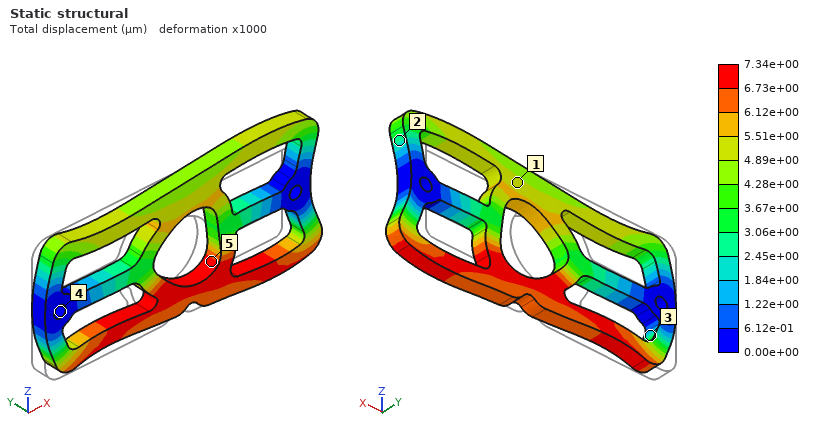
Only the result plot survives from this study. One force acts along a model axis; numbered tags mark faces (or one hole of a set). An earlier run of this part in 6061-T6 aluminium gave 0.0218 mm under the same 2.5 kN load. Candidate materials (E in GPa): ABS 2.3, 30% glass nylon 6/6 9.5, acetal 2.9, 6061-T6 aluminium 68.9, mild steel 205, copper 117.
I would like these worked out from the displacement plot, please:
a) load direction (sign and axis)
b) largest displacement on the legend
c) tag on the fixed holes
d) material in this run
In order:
+X
7.34e+00 µm
4
mild steel
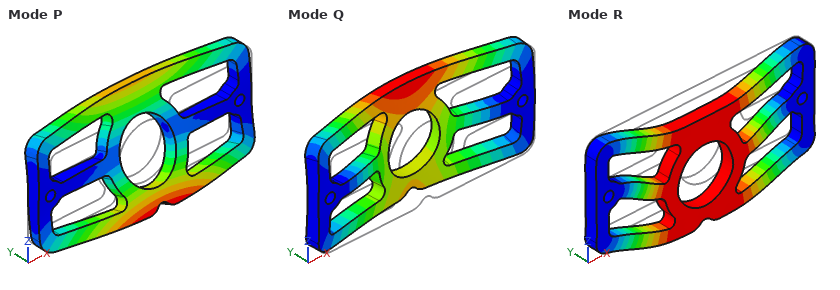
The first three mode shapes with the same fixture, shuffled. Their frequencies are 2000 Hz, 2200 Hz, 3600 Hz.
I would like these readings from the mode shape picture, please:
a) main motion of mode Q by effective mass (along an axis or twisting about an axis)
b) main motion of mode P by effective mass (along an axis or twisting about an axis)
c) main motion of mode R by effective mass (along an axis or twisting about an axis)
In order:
along Y
twisting about X
along Z
